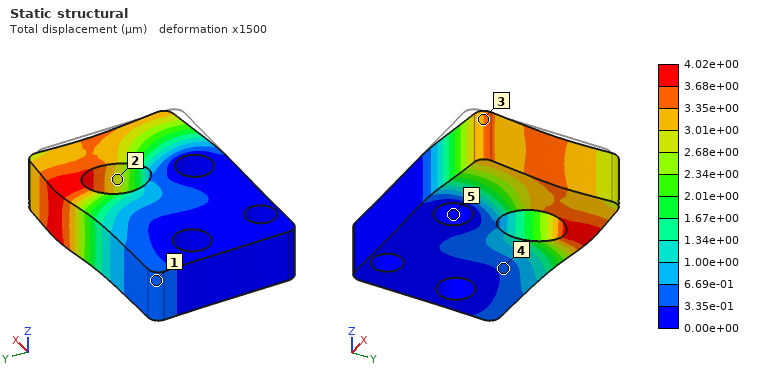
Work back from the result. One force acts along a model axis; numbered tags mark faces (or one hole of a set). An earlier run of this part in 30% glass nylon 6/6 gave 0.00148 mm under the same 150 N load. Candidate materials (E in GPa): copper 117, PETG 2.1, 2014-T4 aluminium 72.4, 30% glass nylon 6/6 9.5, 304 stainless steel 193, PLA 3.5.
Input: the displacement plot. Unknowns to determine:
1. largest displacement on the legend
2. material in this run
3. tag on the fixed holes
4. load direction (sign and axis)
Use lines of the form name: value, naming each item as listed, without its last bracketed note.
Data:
largest displacement on the legend: 4.02e+00 µm
material in this run: PLA
tag on the fixed holes: 5
load direction: +Y
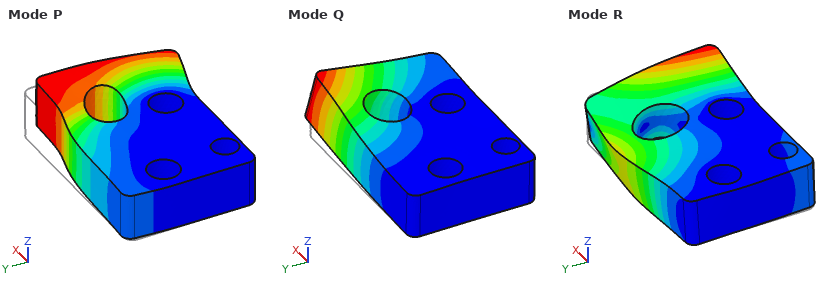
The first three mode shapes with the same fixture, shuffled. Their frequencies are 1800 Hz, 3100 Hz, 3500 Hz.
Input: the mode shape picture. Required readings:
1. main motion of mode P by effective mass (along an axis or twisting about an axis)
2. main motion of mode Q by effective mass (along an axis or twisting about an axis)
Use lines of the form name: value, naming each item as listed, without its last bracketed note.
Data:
main motion of mode P by effective mass: along Y
main motion of mode Q by effective mass: along Z
